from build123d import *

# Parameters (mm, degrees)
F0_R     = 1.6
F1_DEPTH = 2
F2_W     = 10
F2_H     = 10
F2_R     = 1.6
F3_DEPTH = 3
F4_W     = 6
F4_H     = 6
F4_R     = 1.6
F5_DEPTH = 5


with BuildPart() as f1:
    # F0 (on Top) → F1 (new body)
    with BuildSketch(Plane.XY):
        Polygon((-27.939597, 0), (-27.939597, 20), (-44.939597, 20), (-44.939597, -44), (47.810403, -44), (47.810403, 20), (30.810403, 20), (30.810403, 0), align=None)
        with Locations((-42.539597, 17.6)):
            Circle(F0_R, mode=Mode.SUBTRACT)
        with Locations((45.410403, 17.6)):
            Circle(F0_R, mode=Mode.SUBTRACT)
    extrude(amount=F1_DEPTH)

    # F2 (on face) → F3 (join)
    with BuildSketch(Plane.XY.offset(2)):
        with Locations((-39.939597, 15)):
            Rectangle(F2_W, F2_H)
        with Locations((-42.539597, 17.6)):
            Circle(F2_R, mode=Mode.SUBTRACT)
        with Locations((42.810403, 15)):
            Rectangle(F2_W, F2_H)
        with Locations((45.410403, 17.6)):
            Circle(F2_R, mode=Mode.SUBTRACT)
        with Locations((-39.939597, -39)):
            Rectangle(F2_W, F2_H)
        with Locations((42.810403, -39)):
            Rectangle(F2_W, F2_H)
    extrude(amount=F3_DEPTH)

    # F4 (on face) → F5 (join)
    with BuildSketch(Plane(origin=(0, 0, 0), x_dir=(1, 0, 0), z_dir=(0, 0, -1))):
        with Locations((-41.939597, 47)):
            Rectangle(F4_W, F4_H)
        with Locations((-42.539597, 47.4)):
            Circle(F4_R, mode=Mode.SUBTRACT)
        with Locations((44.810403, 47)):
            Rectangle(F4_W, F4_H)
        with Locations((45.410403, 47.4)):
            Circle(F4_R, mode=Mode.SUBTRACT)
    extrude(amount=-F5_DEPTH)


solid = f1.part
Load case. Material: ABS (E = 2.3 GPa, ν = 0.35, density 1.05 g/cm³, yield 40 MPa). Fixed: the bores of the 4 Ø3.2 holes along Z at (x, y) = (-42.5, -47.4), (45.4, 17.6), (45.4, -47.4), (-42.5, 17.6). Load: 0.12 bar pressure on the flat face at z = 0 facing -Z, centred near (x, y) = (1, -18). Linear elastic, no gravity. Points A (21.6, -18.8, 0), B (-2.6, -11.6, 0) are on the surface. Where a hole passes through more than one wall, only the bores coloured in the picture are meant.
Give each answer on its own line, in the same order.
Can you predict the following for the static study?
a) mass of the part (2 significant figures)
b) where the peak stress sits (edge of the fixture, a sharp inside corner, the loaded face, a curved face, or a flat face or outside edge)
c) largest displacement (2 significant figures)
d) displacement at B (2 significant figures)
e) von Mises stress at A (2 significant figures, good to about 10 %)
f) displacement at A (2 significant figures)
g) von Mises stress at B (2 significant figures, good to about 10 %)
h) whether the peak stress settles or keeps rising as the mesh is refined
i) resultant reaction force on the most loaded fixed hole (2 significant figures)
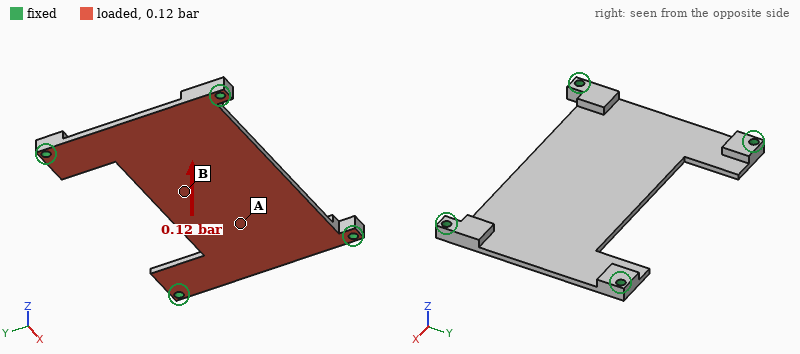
11 g
edge of the fixture
1.3 mm
1.2 mm
2.5 MPa
0.82 mm
5.0 MPa
keeps rising
35 N
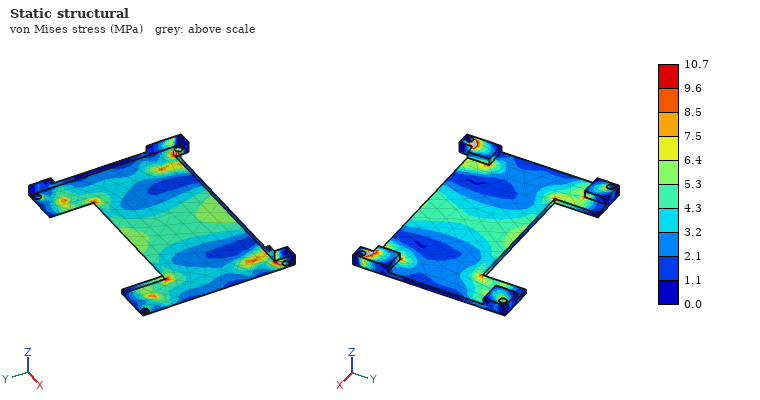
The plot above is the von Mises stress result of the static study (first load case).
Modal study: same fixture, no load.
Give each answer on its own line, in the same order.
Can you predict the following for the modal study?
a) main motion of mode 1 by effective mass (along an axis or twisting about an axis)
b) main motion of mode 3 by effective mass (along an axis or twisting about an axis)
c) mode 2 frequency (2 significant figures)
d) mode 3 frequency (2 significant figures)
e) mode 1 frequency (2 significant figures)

along Z
twisting about Y
730 Hz
940 Hz
400 Hz
